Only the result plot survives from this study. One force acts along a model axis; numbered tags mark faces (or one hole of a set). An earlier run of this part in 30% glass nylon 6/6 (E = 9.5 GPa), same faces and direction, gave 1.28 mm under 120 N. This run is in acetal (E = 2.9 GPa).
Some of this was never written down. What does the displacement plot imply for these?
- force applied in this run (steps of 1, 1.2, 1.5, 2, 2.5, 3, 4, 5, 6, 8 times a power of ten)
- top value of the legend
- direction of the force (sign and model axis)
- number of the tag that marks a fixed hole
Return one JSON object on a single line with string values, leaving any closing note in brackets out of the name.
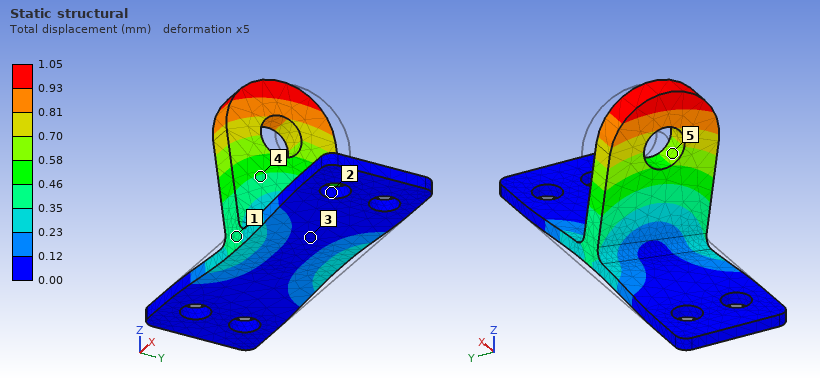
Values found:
{"force applied in this run": "30 N", "top value of the legend": "1.05 mm", "direction of the force": "-Y", "number of the tag that marks a fixed hole": "2"}
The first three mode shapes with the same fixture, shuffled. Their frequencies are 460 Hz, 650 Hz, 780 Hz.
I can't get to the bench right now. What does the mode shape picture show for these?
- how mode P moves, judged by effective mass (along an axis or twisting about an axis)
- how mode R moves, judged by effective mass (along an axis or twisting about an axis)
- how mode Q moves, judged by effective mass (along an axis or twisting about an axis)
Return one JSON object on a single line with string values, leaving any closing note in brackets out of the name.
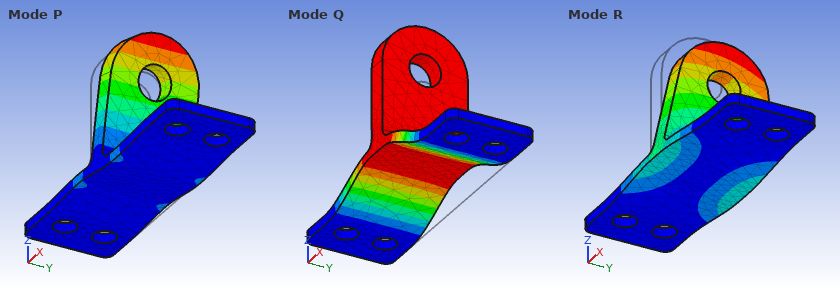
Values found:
{"how mode P moves, judged by effective mass": "along X", "how mode R moves, judged by effective mass": "along Y", "how mode Q moves, judged by effective mass": "along Z"}
